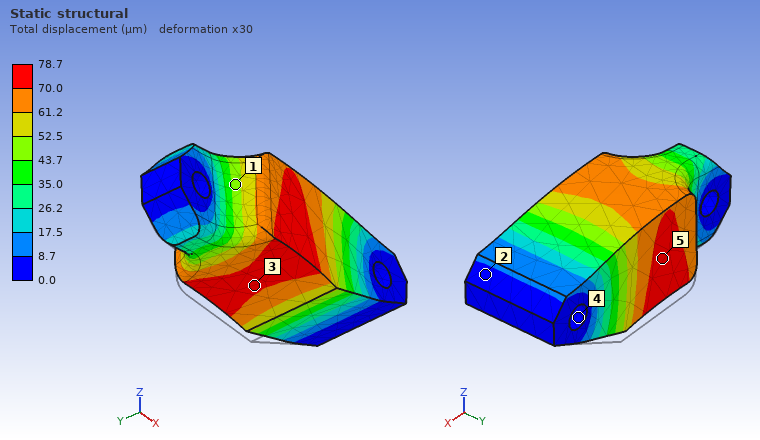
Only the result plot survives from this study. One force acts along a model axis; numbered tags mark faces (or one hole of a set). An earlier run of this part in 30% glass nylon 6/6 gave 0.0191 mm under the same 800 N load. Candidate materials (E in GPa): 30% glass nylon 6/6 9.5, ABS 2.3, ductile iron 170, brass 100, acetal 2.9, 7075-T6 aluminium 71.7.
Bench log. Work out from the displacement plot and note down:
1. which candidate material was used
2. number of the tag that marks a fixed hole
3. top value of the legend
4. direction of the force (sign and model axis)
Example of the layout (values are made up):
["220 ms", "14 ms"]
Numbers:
["ABS", "4", "78.7 µm", "+Z"]
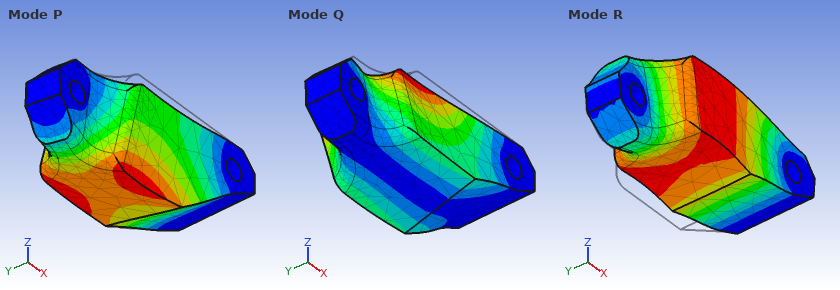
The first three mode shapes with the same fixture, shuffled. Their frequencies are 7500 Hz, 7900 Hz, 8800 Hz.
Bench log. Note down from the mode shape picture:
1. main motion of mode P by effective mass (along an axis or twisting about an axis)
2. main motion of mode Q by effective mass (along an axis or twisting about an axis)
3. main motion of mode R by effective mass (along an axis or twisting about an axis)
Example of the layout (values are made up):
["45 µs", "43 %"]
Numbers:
["along Y", "along Y", "along Z"]
